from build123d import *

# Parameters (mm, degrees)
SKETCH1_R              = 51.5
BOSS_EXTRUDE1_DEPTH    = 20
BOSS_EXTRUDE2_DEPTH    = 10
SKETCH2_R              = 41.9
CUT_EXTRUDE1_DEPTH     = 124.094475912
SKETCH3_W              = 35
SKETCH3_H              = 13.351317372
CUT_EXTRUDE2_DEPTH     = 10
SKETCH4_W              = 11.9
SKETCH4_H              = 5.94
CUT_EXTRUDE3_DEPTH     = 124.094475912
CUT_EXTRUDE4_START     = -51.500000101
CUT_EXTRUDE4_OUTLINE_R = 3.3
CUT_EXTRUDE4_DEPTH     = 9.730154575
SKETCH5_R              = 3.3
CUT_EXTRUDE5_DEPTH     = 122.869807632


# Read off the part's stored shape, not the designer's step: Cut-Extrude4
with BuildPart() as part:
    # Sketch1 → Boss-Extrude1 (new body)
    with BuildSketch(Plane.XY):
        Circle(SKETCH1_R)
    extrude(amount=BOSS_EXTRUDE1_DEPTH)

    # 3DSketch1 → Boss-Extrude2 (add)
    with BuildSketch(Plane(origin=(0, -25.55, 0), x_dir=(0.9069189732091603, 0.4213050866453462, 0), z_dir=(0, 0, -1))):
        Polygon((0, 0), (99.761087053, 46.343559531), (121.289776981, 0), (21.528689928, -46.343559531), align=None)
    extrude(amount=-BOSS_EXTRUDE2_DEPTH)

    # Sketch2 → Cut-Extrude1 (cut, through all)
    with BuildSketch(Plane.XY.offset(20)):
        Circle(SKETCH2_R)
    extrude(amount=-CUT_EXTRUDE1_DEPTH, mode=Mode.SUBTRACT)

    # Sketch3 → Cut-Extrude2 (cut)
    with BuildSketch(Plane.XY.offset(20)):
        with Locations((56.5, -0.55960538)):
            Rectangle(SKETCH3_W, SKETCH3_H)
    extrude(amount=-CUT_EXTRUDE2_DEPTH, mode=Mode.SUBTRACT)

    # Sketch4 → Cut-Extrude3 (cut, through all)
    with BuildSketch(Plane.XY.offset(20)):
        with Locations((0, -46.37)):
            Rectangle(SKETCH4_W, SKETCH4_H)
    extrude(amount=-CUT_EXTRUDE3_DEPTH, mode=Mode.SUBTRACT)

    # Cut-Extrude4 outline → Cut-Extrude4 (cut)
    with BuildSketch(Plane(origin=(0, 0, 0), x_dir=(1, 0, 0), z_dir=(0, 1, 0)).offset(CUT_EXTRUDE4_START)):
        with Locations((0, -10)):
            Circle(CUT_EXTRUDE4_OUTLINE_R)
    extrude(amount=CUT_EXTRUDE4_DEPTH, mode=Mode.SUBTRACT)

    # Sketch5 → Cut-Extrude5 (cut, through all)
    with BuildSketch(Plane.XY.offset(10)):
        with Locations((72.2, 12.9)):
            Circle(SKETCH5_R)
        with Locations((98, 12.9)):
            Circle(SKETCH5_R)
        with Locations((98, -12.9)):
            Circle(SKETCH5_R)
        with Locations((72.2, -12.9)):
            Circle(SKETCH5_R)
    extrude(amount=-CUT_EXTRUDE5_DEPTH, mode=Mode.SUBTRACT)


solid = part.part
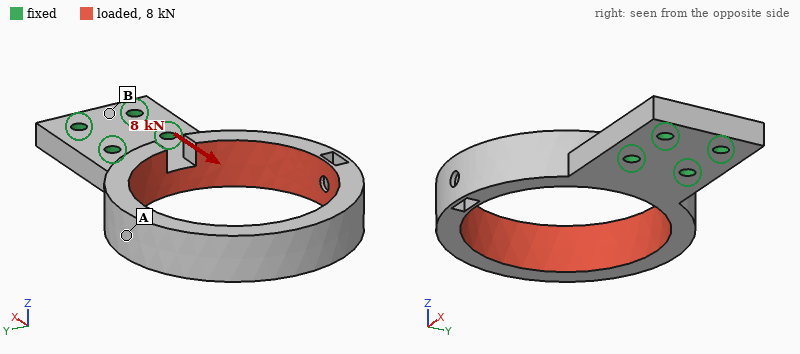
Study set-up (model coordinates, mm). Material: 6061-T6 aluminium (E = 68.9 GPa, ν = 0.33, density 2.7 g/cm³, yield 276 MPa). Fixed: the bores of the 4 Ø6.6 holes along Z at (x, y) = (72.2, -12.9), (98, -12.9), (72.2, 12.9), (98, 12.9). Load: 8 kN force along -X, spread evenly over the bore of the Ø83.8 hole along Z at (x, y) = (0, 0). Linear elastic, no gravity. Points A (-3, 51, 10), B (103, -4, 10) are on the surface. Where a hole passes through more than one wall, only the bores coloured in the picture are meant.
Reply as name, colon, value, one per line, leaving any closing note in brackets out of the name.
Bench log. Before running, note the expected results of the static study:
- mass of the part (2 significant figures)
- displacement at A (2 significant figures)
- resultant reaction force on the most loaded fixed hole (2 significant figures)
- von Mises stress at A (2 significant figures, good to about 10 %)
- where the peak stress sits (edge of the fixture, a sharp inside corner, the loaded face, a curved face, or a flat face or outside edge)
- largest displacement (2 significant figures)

mass of the part: 220 g
displacement at A: 0.37 mm
resultant reaction force on the most loaded fixed hole: 3.7 kN
von Mises stress at A: 65 MPa
where the peak stress sits: the loaded face
largest displacement: 0.65 mm
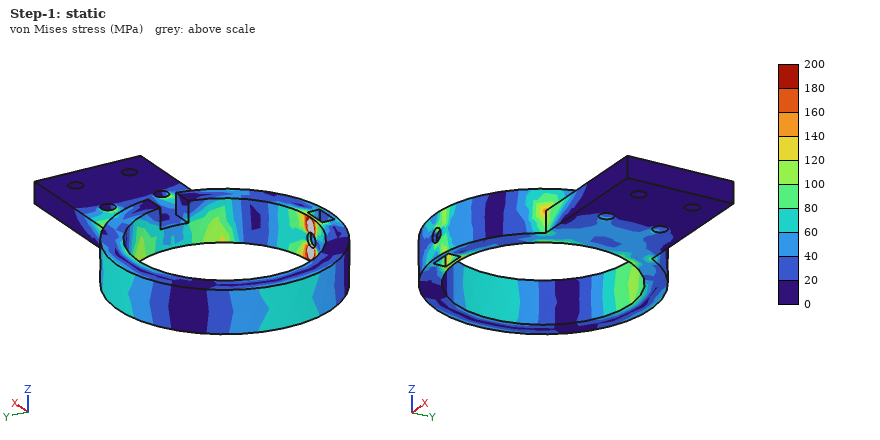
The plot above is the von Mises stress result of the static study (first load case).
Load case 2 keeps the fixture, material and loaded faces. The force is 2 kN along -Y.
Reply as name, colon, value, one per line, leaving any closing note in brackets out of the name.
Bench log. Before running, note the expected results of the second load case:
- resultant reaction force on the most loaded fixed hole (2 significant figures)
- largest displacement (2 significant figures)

resultant reaction force on the most loaded fixed hole: 3.9 kN
largest displacement: 0.69 mm
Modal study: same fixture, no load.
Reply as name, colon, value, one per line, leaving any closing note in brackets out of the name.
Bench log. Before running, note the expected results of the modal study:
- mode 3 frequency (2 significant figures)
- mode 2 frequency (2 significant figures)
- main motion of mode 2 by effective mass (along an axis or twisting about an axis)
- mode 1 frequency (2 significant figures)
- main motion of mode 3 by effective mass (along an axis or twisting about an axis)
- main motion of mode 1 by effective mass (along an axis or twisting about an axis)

mode 3 frequency: 1200 Hz
mode 2 frequency: 780 Hz
main motion of mode 2 by effective mass: along Y
mode 1 frequency: 500 Hz
main motion of mode 3 by effective mass: twisting about X
main motion of mode 1 by effective mass: along Z
